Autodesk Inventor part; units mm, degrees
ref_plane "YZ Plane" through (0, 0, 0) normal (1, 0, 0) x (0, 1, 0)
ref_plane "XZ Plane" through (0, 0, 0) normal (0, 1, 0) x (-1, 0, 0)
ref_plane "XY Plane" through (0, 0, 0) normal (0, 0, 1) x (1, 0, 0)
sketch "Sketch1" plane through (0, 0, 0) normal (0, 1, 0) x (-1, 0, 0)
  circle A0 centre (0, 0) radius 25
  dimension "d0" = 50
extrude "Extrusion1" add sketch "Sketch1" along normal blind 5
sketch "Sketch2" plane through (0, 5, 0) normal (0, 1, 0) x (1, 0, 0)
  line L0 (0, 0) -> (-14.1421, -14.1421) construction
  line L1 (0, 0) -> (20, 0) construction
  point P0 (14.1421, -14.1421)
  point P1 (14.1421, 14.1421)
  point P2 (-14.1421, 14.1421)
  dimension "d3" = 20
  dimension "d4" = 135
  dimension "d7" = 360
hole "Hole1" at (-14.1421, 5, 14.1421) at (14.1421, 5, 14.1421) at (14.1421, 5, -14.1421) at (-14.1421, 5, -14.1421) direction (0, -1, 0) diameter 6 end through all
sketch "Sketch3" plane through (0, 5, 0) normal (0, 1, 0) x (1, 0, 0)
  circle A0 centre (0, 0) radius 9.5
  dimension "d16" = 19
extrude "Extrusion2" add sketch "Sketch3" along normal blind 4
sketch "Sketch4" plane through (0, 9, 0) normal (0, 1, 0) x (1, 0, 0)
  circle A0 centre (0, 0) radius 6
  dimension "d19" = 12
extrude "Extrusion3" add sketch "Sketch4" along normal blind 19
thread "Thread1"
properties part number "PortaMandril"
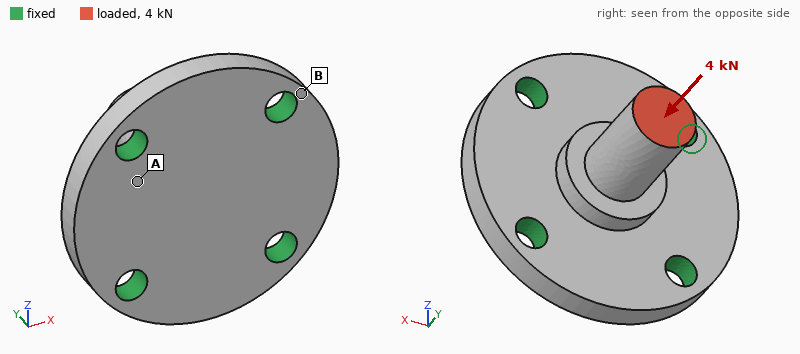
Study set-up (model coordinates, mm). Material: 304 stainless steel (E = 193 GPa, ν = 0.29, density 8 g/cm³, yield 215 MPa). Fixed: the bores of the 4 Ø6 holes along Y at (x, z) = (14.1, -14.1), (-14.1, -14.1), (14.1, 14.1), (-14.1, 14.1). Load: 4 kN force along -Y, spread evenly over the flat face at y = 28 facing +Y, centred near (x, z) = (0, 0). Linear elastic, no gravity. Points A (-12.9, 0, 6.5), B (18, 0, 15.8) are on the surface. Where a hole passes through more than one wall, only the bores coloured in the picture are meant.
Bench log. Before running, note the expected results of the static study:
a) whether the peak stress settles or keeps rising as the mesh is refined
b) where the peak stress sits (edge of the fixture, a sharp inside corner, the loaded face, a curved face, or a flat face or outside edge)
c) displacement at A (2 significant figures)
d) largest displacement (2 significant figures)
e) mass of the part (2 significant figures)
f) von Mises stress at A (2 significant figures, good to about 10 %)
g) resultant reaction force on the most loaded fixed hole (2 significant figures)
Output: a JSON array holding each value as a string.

["keeps rising", "edge of the fixture", "2.6 µm", "10 µm", "100 g", "22 MPa", "1.1 kN"]
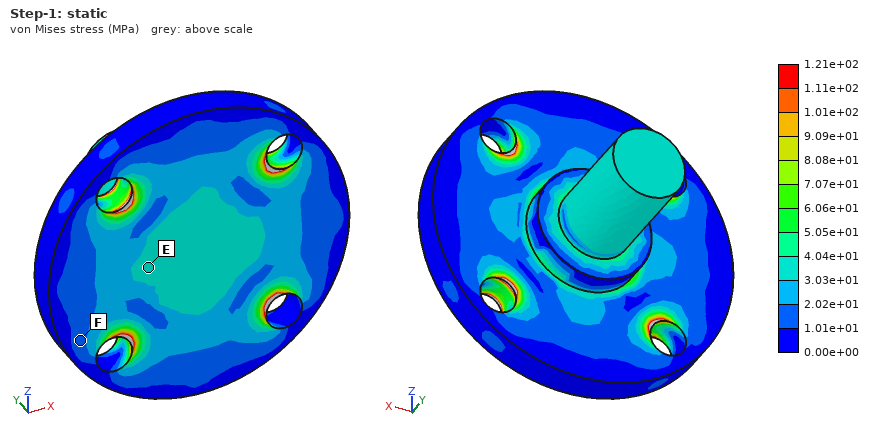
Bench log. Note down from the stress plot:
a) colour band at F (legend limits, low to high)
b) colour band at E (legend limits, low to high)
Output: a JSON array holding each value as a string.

["1.01e+01 to 2.02e+01 MPa", "3.03e+01 to 4.04e+01 MPa"]
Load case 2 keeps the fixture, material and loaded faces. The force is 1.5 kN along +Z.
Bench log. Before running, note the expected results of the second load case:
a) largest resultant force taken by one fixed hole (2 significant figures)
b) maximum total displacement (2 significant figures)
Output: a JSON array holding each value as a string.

["920 N", "44 µm"]
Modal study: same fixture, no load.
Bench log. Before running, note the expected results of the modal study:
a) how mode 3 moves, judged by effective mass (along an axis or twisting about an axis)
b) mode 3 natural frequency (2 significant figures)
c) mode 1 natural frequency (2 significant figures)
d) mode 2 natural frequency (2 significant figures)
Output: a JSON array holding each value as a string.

["along Y", "19 kHz", "12 kHz", "12 kHz"]
